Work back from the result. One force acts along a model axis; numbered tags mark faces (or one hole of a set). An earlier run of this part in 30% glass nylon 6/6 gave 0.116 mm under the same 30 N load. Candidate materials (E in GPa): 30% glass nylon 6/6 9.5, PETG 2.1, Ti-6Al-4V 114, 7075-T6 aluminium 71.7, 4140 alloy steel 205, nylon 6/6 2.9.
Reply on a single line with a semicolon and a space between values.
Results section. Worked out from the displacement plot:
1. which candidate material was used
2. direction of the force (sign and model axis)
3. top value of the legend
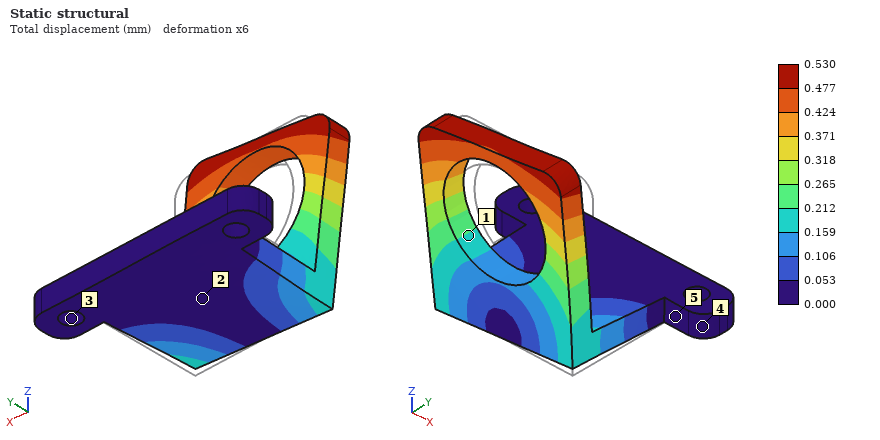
PETG; -X; 0.530 mm
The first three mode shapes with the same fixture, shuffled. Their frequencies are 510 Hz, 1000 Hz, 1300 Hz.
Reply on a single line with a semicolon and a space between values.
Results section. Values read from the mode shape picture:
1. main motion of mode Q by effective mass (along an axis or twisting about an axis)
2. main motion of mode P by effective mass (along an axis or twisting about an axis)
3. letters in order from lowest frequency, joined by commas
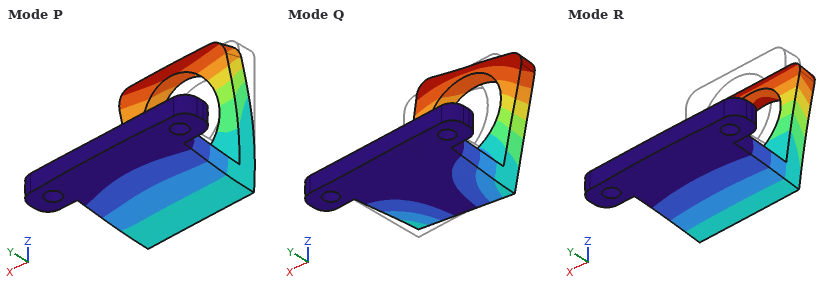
along X; along Z; R, Q, P
